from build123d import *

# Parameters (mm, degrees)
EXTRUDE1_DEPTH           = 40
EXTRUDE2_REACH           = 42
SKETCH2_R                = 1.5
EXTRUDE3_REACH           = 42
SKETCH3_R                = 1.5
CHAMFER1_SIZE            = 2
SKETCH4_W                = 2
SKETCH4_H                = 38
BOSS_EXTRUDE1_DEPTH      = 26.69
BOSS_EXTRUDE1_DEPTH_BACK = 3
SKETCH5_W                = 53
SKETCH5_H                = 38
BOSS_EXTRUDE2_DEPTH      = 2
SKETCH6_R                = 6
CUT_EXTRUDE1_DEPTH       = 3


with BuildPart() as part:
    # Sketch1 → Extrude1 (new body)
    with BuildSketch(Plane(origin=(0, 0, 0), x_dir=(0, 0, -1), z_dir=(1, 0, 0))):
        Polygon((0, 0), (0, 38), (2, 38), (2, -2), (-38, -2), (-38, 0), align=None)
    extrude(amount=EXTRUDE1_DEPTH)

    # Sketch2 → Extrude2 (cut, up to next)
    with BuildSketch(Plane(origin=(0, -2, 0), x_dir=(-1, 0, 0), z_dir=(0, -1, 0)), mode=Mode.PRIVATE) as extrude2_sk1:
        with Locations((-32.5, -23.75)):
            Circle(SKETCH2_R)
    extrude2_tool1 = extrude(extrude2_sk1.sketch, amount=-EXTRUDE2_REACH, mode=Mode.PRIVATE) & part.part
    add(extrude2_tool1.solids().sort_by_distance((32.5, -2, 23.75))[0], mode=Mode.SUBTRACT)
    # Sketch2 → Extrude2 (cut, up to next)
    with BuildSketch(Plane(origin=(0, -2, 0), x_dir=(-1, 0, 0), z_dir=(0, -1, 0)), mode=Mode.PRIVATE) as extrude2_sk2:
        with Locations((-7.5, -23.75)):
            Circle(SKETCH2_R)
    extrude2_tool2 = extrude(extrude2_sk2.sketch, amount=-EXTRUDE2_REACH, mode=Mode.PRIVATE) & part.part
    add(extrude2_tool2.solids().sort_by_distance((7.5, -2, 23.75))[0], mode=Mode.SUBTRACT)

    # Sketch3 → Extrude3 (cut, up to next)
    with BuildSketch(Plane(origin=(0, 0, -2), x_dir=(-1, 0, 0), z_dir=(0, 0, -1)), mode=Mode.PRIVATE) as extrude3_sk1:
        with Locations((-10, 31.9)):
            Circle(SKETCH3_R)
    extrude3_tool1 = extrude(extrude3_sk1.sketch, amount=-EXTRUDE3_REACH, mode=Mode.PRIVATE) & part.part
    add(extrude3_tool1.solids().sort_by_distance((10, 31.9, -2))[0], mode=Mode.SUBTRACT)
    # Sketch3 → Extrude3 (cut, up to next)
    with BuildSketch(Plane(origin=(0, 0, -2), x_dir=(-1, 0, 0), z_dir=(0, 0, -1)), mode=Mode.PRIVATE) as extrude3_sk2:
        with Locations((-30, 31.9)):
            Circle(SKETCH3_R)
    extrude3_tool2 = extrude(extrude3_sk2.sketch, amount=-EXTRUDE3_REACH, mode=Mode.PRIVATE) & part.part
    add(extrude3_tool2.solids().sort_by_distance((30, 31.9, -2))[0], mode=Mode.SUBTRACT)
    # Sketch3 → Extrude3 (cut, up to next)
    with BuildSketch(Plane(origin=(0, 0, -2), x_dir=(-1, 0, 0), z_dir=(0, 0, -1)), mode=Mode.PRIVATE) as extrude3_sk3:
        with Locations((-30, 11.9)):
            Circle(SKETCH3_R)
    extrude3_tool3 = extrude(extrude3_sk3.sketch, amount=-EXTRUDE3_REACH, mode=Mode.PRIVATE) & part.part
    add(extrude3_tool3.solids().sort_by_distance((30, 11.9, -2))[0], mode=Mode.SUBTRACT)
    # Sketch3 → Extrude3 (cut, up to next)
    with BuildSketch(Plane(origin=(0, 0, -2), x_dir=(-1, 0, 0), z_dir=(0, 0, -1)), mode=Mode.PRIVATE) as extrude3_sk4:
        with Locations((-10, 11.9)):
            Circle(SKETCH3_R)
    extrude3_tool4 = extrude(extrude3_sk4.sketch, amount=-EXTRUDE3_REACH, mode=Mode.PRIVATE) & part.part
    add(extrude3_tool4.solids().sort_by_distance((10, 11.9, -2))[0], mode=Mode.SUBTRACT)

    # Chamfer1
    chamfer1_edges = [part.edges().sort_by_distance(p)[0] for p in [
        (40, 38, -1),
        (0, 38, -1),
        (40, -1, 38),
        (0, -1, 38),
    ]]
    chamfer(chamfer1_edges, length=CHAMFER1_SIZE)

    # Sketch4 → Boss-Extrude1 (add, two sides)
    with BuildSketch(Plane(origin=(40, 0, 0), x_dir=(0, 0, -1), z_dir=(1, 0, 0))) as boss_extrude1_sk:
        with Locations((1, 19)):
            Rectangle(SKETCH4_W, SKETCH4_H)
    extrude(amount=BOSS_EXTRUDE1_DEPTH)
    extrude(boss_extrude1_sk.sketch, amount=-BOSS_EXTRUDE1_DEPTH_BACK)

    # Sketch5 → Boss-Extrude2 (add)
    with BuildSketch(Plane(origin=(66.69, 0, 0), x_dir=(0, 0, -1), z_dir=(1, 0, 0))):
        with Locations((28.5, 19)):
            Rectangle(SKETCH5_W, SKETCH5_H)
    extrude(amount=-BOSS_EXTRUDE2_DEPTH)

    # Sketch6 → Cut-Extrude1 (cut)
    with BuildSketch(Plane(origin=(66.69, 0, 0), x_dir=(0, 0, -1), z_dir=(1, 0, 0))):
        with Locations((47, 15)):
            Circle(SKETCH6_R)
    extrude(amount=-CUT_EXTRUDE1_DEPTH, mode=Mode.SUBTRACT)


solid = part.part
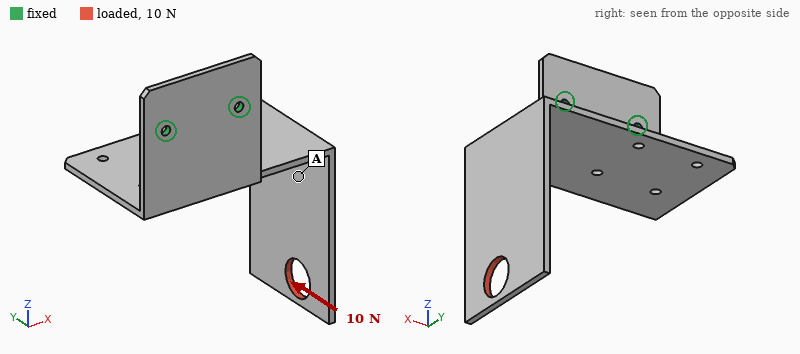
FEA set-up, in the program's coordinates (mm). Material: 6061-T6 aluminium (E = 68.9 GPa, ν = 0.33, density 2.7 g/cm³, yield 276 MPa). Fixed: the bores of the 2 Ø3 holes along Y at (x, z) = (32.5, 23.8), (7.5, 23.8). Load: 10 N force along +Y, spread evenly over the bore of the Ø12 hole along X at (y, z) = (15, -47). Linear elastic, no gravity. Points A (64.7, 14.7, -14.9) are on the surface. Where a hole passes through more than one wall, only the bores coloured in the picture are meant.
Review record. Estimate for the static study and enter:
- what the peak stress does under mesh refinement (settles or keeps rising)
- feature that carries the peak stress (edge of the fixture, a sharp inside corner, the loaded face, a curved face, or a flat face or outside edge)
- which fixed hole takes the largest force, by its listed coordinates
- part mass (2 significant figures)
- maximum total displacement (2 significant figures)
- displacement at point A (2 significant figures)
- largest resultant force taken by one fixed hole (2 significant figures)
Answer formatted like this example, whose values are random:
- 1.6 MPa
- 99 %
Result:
- keeps rising
- edge of the fixture
- (32.5, 23.8)
- 32 g
- 1.2 mm
- 0.48 mm
- 21 N
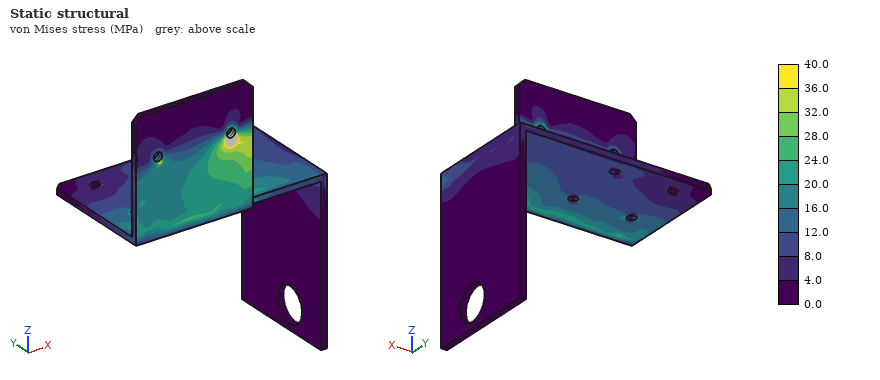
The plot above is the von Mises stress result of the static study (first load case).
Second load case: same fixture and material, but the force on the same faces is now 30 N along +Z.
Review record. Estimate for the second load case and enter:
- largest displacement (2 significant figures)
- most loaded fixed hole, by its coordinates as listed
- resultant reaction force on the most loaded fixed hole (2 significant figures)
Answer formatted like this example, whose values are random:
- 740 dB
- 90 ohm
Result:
- 1.3 mm
- (32.5, 23.8)
- 68 N
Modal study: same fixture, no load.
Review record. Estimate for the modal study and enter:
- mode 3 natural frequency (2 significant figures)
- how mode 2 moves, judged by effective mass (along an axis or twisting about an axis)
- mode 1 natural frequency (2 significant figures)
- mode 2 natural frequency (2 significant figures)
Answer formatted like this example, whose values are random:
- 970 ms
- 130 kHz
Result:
- 560 Hz
- along X
- 180 Hz
- 280 Hz
